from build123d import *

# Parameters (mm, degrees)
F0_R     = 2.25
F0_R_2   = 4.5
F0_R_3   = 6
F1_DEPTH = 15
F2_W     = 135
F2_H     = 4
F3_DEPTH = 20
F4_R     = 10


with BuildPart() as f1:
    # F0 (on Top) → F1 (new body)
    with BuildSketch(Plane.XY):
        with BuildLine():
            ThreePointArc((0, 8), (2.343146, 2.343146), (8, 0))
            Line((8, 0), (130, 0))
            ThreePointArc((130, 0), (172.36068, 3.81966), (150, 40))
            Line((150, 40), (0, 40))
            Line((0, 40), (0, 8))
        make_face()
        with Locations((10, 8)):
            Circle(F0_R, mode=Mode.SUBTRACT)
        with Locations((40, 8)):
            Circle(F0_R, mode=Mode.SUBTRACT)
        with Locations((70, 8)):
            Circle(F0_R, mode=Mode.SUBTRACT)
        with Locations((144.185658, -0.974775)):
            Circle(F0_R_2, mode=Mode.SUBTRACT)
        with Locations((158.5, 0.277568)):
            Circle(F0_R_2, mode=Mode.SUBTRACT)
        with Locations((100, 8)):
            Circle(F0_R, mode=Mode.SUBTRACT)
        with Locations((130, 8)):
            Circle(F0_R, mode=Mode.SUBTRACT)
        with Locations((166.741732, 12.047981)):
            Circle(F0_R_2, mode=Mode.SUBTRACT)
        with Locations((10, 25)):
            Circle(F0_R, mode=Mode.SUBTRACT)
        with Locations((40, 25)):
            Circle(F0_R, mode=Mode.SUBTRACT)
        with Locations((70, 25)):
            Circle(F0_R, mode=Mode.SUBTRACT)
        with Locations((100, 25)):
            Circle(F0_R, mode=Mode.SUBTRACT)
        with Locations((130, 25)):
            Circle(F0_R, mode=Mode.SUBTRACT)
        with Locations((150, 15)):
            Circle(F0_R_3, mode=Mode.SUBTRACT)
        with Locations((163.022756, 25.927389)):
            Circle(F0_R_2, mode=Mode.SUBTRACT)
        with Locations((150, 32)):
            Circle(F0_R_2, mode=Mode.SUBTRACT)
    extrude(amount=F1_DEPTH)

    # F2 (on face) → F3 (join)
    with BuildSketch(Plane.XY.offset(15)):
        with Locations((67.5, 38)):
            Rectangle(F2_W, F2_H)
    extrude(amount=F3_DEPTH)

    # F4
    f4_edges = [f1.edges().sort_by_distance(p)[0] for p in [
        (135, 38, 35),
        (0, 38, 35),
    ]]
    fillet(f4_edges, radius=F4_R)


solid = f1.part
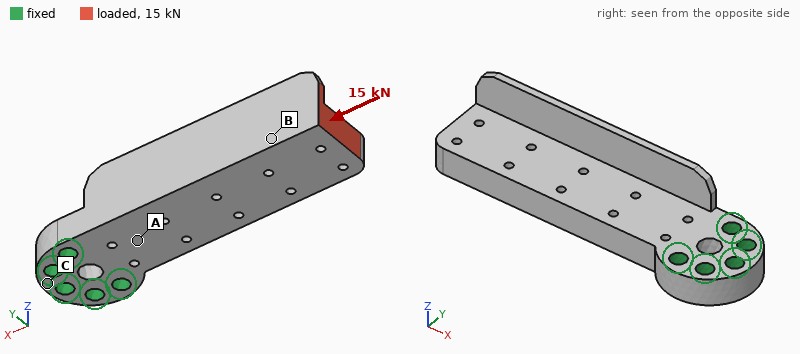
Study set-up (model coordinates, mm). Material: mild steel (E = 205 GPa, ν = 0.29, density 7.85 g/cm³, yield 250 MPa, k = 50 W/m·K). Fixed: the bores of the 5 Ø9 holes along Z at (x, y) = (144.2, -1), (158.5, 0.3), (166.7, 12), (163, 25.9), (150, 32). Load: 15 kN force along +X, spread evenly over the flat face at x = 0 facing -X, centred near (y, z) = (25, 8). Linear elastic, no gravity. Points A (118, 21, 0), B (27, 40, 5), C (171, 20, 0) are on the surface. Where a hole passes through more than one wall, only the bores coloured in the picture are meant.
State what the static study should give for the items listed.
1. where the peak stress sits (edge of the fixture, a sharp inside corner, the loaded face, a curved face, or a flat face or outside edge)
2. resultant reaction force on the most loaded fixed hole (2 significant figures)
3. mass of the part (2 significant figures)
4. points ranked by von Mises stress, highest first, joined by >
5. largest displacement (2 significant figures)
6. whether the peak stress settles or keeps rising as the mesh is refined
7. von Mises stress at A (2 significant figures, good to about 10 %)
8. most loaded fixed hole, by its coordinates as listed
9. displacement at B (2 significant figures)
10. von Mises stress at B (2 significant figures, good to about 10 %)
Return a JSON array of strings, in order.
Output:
["edge of the fixture", "11 kN", "850 g", "B > A > C", "49 µm", "keeps rising", "22 MPa", "(150, 32)", "36 µm", "39 MPa"]
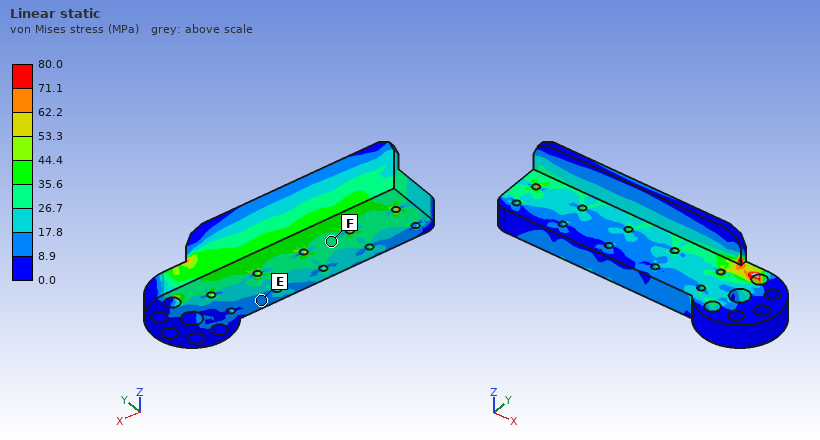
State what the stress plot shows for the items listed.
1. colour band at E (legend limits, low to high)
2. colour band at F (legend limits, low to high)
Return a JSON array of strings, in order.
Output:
["8.9 to 17.8 MPa", "26.7 to 35.6 MPa"]
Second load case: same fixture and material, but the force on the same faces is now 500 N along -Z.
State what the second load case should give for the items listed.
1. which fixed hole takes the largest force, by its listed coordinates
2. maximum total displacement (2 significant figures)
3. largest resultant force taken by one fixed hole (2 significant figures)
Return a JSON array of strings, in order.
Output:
["(144.2, -1)", "0.17 mm", "700 N"]
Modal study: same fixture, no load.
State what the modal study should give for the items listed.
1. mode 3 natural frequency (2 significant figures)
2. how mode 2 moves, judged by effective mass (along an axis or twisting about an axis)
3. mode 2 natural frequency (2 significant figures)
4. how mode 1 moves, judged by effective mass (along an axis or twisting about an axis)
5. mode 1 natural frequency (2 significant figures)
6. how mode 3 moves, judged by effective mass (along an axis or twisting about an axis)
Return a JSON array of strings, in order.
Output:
["2800 Hz", "along Y", "1500 Hz", "along Z", "610 Hz", "twisting about X"]
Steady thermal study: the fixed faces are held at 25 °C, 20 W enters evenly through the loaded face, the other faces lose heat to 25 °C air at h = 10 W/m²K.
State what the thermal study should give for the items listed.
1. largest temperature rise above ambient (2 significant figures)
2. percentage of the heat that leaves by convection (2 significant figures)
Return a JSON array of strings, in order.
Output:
["71 K", "38 %"]
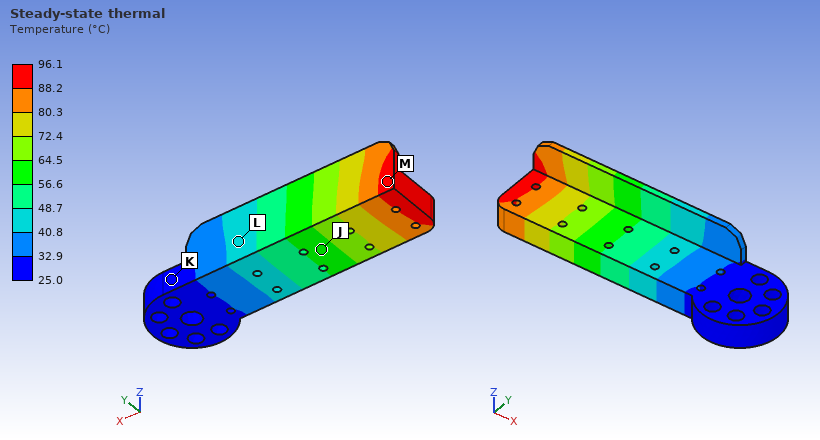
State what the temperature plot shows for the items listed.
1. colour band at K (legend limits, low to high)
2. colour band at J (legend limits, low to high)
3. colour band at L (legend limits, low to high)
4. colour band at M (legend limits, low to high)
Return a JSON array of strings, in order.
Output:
["25.0 to 32.9 °C", "56.6 to 64.5 °C", "40.8 to 48.7 °C", "88.2 to 96.1 °C"]
